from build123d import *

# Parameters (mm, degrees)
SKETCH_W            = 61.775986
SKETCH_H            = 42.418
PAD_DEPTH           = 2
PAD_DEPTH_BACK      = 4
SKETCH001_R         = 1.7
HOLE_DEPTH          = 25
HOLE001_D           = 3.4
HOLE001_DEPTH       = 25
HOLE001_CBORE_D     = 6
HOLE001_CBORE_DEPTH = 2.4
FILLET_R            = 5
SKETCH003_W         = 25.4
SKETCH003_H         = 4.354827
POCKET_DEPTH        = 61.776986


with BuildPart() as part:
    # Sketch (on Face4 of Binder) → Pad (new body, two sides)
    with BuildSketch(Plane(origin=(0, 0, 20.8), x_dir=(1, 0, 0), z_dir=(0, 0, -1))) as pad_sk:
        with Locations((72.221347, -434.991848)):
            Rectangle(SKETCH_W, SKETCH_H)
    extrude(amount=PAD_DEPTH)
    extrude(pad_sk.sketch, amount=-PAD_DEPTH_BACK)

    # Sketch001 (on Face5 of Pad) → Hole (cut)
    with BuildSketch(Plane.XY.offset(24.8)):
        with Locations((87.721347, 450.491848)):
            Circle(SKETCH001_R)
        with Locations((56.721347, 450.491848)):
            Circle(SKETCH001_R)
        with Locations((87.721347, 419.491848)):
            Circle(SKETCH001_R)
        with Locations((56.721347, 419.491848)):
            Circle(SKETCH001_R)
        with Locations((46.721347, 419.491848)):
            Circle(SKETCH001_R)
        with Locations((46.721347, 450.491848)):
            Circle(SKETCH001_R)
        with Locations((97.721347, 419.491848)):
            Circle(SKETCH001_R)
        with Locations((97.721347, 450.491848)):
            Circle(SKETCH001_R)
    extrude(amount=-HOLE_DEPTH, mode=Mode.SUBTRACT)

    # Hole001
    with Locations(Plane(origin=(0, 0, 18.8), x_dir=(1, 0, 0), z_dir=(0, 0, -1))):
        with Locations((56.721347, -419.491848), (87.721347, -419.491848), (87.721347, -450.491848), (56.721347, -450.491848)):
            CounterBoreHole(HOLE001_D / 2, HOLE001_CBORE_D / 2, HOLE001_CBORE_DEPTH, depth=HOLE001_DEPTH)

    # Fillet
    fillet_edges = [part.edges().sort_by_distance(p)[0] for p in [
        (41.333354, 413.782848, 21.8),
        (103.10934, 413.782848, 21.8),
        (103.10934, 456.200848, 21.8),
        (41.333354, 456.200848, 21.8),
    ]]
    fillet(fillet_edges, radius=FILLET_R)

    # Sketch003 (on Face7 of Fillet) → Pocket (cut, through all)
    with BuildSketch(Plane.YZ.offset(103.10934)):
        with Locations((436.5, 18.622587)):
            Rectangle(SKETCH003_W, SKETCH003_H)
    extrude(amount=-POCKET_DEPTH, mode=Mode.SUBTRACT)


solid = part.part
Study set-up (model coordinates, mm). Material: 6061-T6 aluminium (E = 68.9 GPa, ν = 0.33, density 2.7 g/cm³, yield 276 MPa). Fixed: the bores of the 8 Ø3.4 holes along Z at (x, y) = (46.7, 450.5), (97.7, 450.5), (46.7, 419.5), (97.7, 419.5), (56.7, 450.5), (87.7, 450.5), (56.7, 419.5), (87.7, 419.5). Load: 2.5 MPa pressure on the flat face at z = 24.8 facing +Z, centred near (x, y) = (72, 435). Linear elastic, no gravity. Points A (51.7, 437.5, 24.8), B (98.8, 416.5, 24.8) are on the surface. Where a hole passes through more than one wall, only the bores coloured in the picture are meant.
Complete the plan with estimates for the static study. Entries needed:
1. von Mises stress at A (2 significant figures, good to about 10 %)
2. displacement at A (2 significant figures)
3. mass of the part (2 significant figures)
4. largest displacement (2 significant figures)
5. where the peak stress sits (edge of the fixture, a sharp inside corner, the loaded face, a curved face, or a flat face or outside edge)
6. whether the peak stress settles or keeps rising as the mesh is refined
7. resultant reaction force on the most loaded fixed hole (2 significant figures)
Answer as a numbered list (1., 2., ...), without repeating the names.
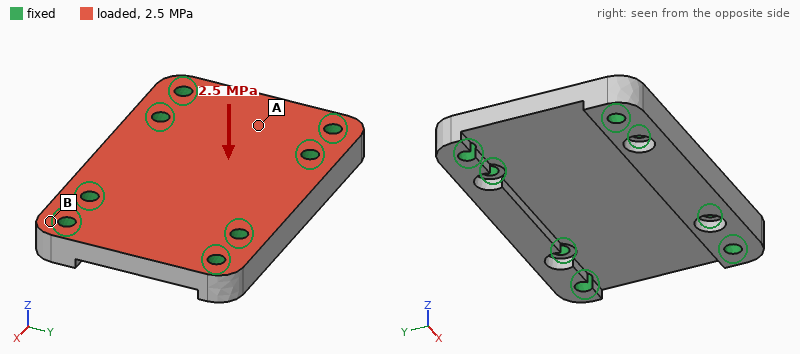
1. 33 MPa
2. 16 µm
3. 32 g
4. 34 µm
5. edge of the fixture
6. keeps rising
7. 1.1 kN
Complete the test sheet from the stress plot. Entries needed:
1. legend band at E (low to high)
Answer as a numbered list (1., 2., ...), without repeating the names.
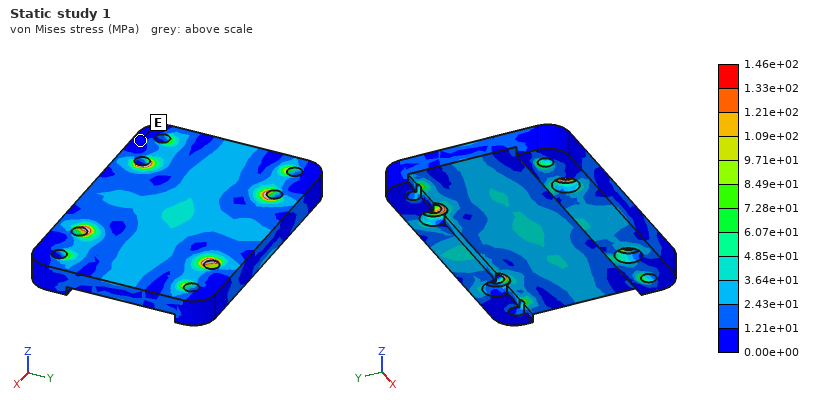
1. 0.00e+00 to 1.21e+01 MPa
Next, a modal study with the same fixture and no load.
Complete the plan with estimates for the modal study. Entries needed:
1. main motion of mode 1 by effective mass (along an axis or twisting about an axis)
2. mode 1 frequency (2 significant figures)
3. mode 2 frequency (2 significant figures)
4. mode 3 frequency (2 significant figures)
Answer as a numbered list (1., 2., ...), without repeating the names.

1. along Z
2. 16 kHz
3. 23 kHz
4. 24 kHz
